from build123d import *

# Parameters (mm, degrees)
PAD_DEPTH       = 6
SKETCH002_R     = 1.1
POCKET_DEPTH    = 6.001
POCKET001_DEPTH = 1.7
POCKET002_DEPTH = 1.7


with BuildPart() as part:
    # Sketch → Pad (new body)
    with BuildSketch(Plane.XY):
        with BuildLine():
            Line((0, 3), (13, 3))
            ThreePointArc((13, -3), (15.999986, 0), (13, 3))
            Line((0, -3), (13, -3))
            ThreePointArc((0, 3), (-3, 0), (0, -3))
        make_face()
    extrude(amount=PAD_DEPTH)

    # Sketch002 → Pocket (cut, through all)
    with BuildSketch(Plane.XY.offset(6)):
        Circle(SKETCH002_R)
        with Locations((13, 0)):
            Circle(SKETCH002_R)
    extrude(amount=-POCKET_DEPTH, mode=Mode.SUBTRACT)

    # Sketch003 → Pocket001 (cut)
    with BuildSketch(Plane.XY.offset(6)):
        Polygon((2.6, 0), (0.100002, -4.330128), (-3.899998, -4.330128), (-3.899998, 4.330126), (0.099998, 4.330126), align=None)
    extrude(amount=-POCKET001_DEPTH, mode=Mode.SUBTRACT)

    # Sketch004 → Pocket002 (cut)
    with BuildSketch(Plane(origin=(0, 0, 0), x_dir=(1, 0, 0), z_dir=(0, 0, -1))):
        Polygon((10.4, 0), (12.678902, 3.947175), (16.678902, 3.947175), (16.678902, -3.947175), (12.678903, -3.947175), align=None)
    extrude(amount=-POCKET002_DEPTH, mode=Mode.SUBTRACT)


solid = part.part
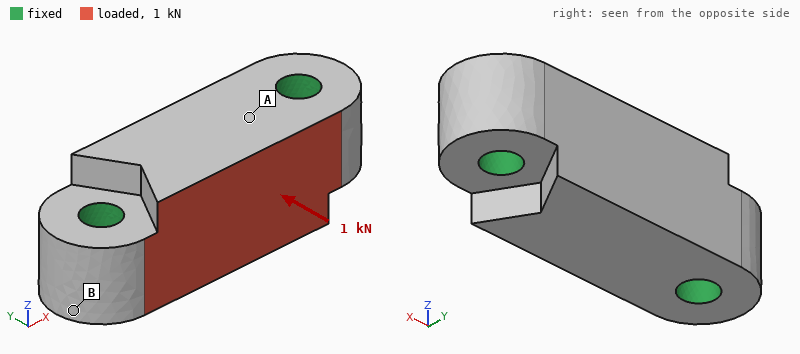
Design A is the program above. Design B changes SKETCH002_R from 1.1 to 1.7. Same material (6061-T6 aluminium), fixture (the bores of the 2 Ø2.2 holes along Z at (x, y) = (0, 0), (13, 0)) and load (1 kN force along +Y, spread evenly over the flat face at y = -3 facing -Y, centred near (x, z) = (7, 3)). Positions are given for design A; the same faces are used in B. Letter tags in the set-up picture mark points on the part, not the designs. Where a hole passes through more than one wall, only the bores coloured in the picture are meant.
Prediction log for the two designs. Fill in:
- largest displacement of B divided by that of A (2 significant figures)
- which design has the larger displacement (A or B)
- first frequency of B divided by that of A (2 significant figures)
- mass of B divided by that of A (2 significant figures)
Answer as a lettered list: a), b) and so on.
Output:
a) 0.79
b) A
c) 1.2
d) 0.91
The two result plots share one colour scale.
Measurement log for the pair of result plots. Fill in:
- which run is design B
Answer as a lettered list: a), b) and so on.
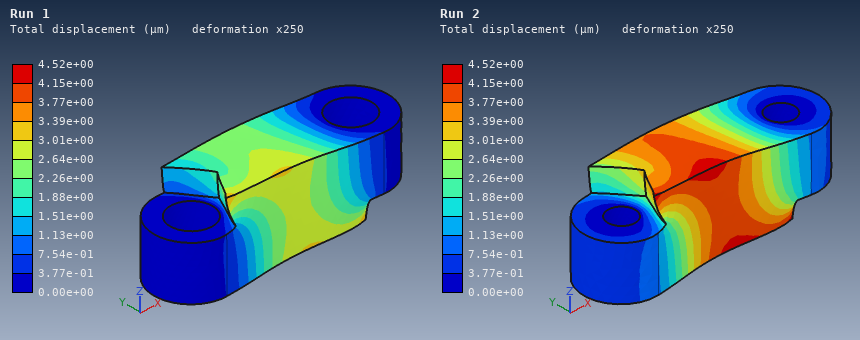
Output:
a) Run 1
